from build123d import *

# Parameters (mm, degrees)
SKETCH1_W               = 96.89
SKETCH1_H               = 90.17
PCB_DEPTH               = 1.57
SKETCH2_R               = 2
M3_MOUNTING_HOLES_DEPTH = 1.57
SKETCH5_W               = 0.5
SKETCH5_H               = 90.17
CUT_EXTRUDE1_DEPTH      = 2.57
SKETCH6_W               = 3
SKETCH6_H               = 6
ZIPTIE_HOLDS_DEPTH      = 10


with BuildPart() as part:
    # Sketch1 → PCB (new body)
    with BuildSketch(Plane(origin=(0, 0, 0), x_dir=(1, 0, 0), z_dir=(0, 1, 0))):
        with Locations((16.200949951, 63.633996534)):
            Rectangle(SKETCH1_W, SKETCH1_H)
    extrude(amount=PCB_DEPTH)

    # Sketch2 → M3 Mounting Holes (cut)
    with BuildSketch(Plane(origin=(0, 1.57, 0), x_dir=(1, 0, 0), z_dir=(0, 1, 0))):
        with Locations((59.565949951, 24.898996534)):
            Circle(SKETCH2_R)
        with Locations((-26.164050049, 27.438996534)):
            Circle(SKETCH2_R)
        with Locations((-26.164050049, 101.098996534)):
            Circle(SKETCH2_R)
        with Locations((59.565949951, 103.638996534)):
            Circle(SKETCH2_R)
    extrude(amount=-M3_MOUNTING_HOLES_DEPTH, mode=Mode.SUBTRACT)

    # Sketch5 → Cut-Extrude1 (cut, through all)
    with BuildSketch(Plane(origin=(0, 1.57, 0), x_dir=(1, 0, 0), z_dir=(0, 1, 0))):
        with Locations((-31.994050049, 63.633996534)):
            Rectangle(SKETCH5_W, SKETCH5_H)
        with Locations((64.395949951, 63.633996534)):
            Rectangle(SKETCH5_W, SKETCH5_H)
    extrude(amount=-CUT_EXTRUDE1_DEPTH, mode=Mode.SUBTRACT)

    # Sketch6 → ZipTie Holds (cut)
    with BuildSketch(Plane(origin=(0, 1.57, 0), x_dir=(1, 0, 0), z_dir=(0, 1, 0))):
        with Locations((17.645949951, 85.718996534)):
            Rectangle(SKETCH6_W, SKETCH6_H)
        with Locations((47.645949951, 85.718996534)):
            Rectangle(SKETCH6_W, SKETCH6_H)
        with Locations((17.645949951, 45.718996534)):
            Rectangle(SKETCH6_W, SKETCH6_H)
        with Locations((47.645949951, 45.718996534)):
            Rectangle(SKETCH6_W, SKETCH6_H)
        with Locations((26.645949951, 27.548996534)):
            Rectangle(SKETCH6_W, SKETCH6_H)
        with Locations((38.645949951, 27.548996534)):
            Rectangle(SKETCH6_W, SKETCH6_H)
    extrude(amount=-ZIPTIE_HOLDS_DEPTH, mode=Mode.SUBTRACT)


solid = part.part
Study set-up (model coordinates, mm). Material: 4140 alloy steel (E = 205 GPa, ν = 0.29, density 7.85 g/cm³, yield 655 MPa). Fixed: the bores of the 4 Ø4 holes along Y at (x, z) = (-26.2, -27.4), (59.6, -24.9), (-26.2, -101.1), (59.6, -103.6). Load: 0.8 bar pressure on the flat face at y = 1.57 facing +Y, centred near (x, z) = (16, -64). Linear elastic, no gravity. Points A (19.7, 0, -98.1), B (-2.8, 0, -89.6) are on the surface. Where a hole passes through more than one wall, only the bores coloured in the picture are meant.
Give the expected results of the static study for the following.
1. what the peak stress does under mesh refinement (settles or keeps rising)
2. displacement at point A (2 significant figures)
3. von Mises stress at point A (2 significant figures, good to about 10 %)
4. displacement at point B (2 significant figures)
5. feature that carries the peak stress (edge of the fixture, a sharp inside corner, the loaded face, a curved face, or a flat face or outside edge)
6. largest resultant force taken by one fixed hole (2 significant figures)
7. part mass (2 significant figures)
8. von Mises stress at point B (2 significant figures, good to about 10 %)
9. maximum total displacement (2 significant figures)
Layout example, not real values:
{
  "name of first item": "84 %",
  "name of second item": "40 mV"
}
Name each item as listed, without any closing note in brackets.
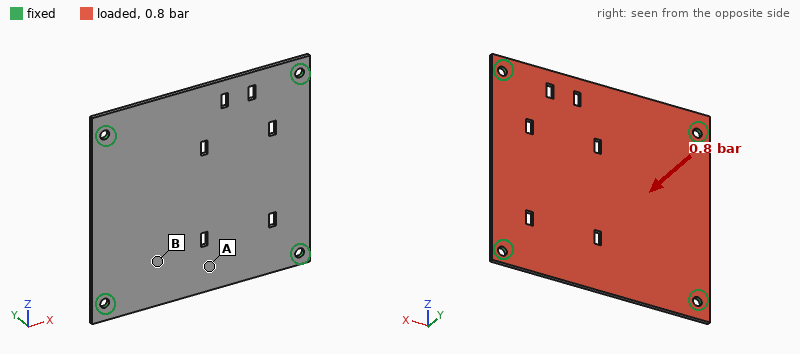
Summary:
{
  "what the peak stress does under mesh refinement": "keeps rising",
  "displacement at point A": "0.26 mm",
  "von Mises stress at point A": "80 MPa",
  "displacement at point B": "0.22 mm",
  "feature that carries the peak stress": "edge of the fixture",
  "largest resultant force taken by one fixed hole": "180 N",
  "part mass": "100 g",
  "von Mises stress at point B": "37 MPa",
  "maximum total displacement": "0.38 mm"
}
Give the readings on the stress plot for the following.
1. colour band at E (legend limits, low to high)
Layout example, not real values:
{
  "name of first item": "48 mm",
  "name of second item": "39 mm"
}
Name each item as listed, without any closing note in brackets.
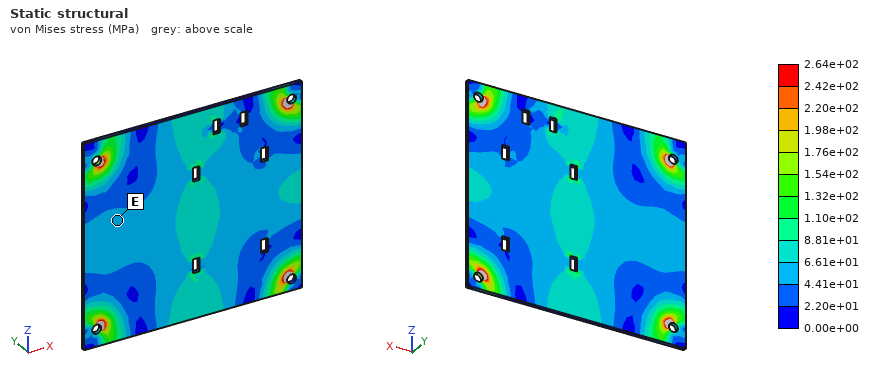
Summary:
{
  "colour band at E": "4.41e+01 to 6.61e+01 MPa"
}
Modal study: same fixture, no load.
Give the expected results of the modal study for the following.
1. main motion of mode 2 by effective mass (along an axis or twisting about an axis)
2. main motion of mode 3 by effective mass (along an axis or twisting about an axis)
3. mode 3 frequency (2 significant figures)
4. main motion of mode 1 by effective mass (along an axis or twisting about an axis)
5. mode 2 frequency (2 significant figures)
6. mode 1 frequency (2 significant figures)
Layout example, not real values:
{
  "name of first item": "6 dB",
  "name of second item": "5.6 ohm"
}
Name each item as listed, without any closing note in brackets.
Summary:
{
  "main motion of mode 2 by effective mass": "twisting about X",
  "main motion of mode 3 by effective mass": "twisting about Z",
  "mode 3 frequency": "1500 Hz",
  "main motion of mode 1 by effective mass": "along Y",
  "mode 2 frequency": "1300 Hz",
  "mode 1 frequency": "800 Hz"
}
